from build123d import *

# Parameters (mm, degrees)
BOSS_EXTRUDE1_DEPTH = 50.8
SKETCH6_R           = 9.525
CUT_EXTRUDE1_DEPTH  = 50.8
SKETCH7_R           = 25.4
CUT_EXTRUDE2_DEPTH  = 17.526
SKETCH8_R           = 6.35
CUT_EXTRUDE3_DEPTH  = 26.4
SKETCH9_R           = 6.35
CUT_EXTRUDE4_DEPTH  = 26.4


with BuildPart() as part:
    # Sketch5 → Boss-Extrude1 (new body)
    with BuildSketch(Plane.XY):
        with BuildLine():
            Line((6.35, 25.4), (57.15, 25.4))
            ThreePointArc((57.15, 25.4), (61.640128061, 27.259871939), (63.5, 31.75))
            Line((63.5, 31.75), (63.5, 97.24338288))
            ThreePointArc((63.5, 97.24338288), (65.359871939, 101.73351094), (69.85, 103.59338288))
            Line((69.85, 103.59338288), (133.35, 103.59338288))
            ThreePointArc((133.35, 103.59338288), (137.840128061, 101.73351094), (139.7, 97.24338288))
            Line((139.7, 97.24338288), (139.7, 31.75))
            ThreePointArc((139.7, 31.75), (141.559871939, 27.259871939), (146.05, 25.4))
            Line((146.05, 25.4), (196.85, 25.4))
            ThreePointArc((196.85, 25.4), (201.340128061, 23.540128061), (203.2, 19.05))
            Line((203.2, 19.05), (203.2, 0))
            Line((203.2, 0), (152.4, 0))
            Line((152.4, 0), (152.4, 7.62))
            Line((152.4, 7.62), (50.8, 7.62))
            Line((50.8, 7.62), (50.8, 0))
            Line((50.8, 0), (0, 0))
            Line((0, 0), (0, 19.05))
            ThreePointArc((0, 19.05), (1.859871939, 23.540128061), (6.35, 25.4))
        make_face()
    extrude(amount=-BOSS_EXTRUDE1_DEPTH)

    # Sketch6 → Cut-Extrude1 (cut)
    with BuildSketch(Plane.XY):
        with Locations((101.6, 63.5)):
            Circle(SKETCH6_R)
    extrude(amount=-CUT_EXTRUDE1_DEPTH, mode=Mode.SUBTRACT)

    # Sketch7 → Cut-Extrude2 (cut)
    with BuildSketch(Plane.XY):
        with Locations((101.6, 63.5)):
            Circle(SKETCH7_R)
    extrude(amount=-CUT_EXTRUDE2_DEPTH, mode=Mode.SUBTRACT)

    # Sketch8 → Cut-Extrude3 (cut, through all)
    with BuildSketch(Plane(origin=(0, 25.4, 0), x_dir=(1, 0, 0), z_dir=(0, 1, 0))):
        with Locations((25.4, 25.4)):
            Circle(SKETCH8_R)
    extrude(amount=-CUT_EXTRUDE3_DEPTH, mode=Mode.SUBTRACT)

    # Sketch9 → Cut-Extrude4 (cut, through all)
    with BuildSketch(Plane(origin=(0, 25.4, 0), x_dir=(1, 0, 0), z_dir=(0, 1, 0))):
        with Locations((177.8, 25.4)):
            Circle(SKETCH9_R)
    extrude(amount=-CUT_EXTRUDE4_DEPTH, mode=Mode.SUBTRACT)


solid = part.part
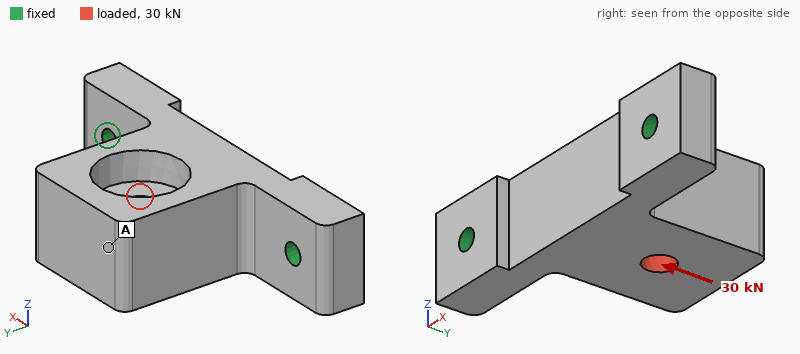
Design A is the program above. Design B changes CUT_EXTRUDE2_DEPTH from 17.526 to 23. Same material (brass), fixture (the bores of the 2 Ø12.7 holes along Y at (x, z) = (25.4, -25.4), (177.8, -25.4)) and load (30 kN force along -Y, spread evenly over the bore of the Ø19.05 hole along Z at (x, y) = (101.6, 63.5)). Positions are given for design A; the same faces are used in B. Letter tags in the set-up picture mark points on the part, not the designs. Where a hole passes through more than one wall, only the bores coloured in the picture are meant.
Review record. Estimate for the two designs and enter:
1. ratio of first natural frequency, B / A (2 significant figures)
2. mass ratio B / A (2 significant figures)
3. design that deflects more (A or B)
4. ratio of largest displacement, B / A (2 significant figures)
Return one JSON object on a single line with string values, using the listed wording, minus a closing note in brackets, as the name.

{"ratio of first natural frequency, B / A": "1.0", "mass ratio B / A": "0.98", "design that deflects more": "B", "ratio of largest displacement, B / A": "1.2"}
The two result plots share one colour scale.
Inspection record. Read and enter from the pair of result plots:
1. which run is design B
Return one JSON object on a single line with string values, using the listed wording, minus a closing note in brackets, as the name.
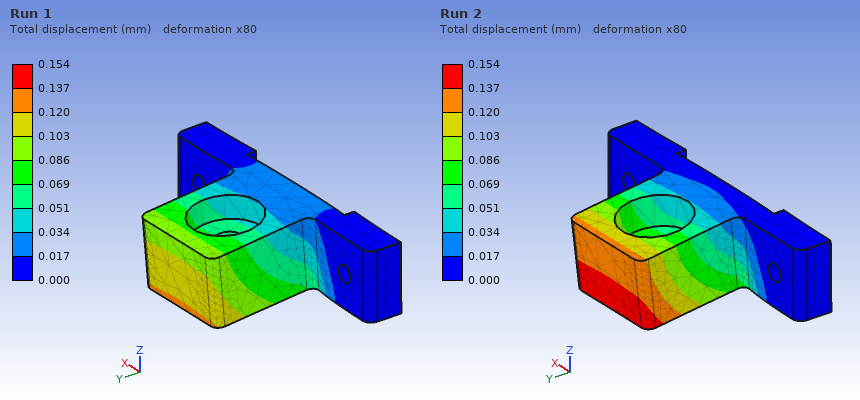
{"which run is design B": "Run 2"}
